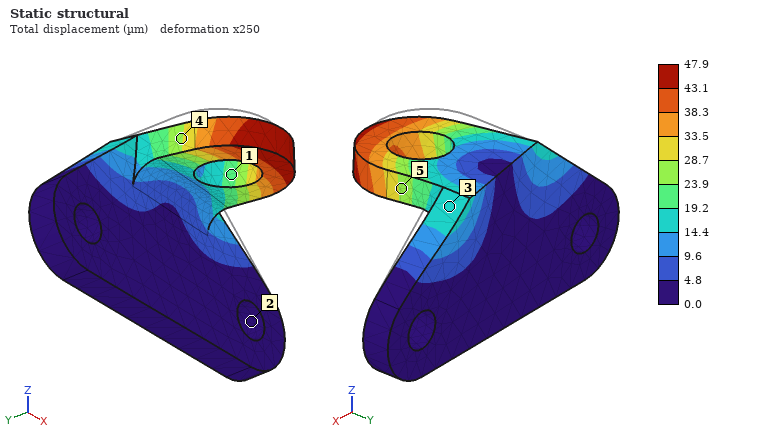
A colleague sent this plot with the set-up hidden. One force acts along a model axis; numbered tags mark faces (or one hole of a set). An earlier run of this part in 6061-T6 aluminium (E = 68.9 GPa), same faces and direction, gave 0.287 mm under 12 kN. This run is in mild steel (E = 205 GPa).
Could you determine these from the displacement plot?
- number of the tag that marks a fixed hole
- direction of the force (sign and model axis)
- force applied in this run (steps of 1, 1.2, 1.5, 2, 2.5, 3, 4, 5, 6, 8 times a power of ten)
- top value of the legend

2
+X
6 kN
47.9 µm
